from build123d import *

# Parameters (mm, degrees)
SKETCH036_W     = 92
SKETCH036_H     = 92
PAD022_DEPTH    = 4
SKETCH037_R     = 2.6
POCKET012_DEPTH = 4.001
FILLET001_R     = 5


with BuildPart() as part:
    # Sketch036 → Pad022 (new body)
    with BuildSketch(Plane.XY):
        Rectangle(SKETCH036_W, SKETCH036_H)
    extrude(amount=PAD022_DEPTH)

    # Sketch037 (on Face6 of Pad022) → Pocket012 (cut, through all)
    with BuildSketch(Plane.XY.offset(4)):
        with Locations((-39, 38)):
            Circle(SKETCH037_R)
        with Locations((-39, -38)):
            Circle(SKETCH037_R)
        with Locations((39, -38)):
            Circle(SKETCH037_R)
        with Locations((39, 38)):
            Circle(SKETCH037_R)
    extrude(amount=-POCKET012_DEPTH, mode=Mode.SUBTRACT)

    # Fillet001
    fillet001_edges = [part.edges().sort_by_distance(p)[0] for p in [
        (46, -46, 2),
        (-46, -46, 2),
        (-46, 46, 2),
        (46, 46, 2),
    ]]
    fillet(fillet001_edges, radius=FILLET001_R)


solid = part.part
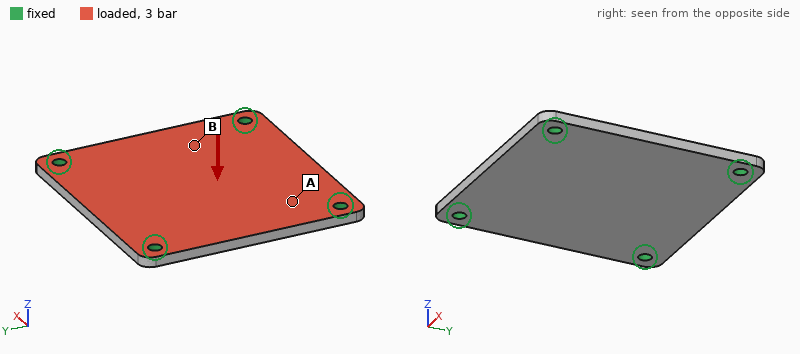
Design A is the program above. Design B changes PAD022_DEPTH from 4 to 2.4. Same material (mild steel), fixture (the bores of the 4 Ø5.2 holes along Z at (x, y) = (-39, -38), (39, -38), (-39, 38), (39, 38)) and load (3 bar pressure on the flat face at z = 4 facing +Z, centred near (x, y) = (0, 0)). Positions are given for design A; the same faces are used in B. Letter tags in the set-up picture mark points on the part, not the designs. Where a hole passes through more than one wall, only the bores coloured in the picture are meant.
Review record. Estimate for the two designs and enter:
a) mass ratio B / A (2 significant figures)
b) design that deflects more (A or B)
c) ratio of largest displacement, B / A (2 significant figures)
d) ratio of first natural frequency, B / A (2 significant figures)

0.60
B
4.4
0.62
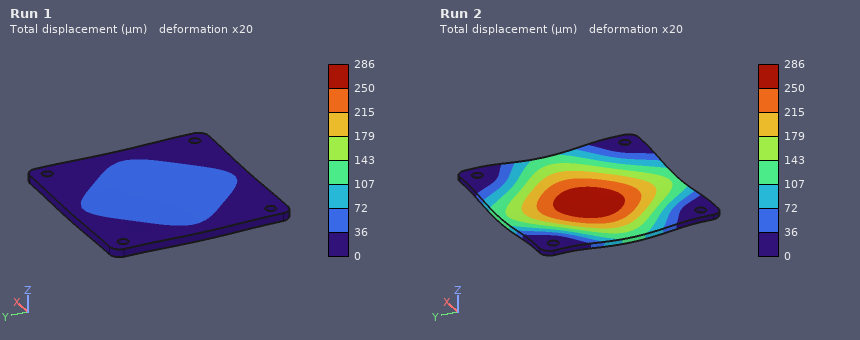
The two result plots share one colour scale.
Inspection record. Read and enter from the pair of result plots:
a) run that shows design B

Run 2
